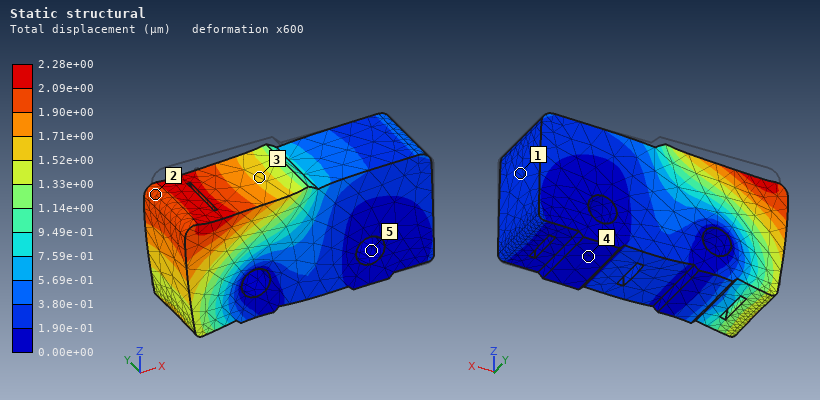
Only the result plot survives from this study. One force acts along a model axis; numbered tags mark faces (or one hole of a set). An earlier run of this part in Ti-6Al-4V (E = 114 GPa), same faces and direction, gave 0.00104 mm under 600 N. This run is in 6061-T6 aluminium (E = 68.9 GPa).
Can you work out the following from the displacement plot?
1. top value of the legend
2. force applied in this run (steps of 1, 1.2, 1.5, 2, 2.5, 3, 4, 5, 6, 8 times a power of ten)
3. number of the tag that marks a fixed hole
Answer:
2.28e+00 µm
800 N
5
